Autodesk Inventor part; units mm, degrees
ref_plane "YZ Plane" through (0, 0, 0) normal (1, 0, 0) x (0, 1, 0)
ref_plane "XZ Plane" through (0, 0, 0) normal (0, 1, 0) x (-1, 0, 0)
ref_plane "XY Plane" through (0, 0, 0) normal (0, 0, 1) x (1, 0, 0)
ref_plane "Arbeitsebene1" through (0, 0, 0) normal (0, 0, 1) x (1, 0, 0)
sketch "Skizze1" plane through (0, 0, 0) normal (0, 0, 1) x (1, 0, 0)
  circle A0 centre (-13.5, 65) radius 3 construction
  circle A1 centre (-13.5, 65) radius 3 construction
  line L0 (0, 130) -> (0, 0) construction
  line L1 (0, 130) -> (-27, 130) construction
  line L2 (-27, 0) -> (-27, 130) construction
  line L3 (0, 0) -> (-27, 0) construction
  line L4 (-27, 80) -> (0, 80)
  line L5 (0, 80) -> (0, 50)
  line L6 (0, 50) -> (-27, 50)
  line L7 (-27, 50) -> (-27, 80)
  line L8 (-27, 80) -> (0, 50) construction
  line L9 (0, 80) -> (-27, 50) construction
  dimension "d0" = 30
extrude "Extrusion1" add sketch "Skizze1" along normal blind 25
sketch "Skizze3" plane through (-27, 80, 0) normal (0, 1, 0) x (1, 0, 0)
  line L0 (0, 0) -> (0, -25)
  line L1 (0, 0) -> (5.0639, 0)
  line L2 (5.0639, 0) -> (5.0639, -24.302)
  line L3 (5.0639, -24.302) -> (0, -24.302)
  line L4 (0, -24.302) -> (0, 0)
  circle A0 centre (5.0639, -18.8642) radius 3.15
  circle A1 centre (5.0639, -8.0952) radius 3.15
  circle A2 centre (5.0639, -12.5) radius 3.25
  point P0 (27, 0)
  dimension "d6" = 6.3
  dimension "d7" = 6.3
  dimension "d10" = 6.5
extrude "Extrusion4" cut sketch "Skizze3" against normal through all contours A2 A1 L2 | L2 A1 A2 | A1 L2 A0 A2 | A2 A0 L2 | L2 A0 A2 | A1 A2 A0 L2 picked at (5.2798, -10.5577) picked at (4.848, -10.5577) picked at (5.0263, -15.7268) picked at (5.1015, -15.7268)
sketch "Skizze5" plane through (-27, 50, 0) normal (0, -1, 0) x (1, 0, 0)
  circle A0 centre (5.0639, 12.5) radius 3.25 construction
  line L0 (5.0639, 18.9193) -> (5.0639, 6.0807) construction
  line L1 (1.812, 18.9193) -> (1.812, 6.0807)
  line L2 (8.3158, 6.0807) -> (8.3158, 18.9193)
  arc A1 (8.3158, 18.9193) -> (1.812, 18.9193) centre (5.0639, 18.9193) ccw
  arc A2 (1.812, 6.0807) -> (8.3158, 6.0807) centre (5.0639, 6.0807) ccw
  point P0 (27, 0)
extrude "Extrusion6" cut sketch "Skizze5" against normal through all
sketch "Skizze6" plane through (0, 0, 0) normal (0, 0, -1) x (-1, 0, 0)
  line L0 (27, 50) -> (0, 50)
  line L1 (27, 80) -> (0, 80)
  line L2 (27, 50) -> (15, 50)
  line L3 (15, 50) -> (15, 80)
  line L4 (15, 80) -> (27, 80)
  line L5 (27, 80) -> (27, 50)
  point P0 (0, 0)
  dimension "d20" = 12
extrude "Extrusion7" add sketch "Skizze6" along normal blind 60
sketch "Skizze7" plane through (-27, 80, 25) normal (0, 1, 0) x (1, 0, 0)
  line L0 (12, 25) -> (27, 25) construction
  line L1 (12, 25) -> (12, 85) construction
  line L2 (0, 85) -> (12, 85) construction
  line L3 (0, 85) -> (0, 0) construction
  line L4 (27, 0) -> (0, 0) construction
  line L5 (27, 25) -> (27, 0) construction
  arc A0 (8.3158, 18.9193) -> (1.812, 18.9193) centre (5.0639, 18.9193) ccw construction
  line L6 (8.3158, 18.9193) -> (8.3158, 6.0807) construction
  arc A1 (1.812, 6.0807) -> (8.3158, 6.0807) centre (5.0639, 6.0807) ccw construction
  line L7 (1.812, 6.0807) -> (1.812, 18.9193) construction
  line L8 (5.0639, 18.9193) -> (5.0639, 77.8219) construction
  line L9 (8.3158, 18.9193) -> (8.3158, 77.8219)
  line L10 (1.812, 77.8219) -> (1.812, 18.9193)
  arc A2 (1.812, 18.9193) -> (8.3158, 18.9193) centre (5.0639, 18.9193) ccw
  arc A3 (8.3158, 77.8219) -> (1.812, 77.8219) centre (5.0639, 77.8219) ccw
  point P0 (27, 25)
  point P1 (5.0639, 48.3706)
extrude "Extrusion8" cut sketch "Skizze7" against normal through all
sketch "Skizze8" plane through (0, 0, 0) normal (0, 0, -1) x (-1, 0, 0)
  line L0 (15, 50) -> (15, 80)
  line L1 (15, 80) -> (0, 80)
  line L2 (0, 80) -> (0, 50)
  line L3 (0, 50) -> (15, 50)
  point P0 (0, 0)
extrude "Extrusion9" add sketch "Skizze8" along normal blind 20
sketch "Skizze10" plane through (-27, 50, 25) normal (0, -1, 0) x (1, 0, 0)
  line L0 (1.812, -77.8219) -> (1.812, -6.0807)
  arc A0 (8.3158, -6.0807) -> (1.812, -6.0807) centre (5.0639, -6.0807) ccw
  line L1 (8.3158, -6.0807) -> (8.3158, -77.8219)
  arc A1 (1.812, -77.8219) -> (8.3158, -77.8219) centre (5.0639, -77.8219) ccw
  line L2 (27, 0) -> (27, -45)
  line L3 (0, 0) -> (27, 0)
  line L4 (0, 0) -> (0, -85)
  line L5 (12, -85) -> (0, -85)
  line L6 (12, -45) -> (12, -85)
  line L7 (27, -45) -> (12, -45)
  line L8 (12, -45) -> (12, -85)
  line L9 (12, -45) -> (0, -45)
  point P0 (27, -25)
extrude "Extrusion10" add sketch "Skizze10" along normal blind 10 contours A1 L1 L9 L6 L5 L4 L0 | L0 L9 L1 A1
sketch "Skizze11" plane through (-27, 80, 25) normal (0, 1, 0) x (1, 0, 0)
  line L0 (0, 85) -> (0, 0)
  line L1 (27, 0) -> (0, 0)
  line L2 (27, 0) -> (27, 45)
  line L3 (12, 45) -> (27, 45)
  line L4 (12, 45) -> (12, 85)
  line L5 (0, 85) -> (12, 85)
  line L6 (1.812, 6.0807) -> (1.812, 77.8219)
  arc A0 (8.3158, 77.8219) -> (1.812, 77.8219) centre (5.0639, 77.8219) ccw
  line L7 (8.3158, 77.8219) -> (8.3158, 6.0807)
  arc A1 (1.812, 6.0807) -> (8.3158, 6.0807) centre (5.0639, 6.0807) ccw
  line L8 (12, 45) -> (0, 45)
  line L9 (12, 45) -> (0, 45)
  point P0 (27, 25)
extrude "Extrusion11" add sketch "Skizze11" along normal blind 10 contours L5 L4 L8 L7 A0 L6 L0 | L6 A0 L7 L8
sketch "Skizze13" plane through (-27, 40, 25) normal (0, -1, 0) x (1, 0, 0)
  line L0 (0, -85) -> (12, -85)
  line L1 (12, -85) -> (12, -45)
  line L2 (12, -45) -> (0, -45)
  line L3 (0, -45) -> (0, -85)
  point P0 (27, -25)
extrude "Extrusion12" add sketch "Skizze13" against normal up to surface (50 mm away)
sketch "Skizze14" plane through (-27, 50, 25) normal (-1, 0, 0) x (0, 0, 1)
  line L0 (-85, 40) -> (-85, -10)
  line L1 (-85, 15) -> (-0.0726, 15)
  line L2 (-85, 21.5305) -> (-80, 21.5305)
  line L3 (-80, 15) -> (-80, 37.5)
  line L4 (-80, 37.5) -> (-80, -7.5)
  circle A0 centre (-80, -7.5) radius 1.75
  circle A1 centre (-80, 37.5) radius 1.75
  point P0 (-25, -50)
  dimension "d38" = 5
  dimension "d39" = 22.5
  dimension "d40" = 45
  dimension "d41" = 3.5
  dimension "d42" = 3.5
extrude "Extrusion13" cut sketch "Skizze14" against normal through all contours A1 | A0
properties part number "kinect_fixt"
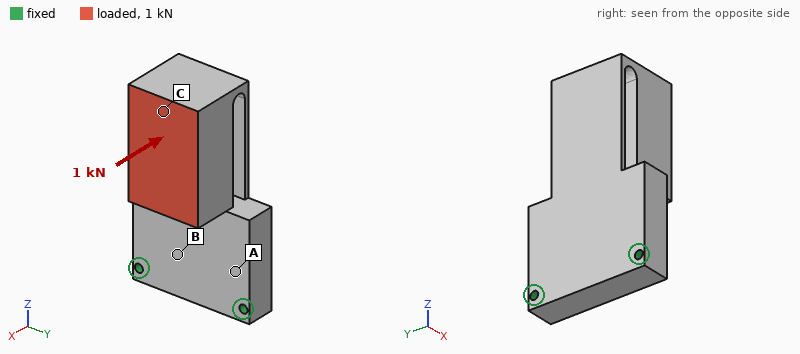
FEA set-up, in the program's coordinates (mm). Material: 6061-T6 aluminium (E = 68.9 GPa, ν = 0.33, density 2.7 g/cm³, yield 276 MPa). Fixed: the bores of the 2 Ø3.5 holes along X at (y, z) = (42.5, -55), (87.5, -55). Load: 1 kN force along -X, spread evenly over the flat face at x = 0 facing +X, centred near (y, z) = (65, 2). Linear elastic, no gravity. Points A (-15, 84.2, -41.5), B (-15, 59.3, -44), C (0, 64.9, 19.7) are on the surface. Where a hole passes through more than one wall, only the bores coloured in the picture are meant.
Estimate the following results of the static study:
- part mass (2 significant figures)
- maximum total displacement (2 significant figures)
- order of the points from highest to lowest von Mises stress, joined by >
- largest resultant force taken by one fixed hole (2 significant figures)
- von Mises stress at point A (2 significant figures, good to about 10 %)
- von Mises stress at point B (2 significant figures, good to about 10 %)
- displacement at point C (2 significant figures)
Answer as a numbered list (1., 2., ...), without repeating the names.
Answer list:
1. 140 g
2. 0.53 mm
3. A > B > C
4. 500 N
5. 44 MPa
6. 29 MPa
7. 0.49 mm
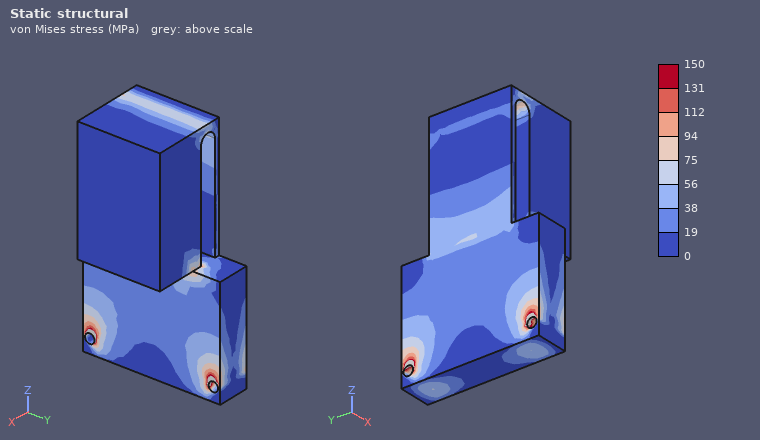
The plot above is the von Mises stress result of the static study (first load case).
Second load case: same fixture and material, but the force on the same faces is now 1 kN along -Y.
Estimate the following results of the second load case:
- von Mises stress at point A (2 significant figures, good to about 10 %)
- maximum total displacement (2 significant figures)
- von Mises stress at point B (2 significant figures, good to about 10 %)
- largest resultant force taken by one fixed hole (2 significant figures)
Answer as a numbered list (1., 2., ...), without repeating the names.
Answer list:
1. 14 MPa
2. 51 µm
3. 13 MPa
4. 1.5 kN
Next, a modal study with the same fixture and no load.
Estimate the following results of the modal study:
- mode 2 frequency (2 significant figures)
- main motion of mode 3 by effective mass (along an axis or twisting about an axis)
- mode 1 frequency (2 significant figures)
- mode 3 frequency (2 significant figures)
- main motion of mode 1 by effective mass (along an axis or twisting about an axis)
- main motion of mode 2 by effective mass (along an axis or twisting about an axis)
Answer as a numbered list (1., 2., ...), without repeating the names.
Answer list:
1. 3600 Hz
2. along X
3. 910 Hz
4. 4700 Hz
5. along X
6. along Y
